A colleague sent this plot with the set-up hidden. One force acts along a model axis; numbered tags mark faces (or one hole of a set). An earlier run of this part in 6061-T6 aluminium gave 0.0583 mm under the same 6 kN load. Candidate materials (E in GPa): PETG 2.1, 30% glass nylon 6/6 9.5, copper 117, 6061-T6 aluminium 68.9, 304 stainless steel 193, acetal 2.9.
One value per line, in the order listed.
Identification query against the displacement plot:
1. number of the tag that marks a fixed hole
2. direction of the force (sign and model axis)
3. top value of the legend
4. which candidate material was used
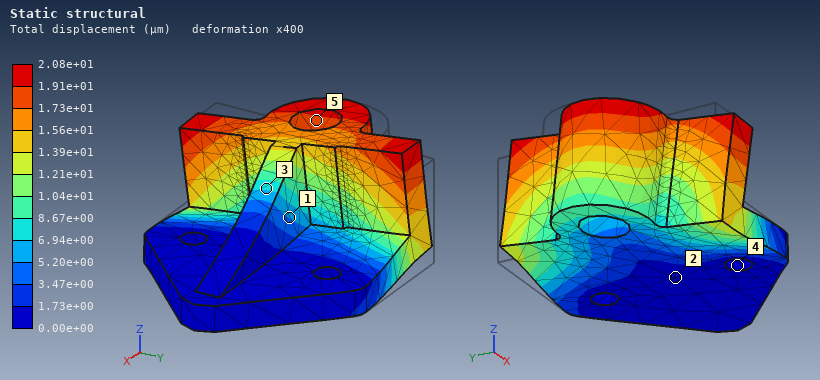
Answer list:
4
-Y
2.08e+01 µm
304 stainless steel
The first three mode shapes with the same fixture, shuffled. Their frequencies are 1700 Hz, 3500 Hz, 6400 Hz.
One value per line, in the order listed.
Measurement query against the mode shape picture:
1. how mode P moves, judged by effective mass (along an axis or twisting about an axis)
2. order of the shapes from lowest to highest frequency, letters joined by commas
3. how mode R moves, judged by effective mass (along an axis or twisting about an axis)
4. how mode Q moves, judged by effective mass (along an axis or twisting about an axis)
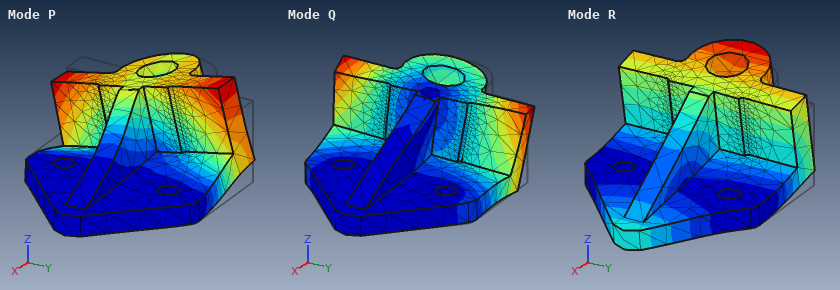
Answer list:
along Y
R, P, Q
along Z
along Y
